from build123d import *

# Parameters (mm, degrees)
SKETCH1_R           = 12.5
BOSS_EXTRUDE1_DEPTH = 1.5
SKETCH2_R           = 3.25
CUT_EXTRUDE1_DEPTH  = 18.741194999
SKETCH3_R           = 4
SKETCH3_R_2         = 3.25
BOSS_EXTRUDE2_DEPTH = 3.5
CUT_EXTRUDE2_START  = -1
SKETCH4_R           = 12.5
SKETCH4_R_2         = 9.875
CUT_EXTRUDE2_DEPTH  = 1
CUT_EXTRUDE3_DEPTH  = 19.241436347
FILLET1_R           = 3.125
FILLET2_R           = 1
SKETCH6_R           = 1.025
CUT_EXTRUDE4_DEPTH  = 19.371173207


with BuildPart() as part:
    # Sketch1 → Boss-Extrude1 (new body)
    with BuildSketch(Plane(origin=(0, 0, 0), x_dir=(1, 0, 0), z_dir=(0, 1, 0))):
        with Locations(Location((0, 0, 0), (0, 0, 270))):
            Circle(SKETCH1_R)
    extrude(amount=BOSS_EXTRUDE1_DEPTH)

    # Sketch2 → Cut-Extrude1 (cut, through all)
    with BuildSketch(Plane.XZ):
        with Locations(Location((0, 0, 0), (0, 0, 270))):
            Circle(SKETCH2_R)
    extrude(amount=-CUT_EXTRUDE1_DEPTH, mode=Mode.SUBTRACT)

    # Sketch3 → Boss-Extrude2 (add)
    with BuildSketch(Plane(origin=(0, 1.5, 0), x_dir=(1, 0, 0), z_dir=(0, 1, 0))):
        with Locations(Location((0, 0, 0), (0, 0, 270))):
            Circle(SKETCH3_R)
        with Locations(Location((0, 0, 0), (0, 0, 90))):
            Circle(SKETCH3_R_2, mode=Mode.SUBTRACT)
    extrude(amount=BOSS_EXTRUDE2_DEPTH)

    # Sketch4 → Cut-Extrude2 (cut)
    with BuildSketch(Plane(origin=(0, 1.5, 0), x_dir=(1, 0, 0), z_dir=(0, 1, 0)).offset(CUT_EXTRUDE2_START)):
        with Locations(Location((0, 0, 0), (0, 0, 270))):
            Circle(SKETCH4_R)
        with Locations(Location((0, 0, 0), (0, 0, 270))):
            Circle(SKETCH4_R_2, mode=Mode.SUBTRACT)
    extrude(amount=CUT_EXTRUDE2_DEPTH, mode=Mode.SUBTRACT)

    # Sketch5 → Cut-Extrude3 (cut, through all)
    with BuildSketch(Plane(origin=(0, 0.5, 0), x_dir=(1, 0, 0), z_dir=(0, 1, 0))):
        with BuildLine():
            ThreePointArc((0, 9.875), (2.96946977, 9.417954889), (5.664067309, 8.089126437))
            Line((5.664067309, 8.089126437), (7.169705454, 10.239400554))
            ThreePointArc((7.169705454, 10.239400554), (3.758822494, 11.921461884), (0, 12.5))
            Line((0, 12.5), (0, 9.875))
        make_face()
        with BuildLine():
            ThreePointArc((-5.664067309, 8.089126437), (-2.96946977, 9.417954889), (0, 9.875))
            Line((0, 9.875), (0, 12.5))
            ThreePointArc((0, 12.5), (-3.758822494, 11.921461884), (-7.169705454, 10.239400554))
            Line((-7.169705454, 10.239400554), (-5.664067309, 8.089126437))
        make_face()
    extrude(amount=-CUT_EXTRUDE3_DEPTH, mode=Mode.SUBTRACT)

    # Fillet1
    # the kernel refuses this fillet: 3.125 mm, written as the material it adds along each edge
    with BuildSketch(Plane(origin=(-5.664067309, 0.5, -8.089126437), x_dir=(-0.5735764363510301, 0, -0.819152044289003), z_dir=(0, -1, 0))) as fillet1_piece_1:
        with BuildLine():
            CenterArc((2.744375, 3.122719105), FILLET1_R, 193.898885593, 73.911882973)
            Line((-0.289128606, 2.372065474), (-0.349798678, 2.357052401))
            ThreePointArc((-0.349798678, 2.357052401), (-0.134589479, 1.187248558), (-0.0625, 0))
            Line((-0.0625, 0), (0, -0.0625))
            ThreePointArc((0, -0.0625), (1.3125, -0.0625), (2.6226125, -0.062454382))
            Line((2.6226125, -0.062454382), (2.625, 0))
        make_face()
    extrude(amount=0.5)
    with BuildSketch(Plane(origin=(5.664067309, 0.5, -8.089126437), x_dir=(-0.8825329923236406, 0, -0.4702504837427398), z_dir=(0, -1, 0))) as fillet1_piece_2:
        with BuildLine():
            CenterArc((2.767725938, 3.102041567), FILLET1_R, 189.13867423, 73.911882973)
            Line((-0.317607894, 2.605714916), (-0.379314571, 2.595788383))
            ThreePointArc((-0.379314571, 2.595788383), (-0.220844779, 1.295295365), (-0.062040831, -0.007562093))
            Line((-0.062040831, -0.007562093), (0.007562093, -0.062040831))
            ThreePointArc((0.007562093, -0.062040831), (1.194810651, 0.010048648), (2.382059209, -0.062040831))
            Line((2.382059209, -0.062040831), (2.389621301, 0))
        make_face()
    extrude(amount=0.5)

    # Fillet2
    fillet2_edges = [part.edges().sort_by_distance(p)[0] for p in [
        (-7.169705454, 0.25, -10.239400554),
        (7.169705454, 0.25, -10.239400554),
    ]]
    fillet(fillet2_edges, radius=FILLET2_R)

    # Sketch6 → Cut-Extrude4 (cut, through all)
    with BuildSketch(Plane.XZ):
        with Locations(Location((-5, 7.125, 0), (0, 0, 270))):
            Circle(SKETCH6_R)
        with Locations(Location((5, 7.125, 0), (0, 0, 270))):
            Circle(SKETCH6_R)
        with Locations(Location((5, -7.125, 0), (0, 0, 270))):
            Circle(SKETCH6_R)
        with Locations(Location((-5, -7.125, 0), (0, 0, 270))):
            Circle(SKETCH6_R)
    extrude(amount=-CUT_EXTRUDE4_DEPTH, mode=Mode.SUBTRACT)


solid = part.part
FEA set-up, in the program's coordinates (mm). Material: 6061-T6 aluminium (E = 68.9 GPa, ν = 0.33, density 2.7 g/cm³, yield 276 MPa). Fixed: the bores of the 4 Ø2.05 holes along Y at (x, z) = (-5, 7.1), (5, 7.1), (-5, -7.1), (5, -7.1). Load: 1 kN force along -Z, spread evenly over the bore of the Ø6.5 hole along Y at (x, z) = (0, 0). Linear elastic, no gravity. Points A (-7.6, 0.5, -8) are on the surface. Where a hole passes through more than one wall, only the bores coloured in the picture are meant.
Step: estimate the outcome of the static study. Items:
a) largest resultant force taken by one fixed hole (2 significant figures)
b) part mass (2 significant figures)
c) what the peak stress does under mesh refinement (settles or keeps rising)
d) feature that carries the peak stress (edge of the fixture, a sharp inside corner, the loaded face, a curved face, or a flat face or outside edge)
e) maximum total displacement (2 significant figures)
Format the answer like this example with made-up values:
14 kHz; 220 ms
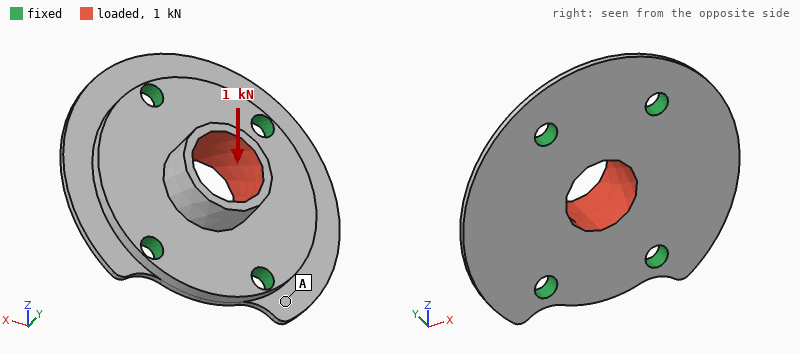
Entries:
270 N; 1.4 g; keeps rising; edge of the fixture; 22 µm
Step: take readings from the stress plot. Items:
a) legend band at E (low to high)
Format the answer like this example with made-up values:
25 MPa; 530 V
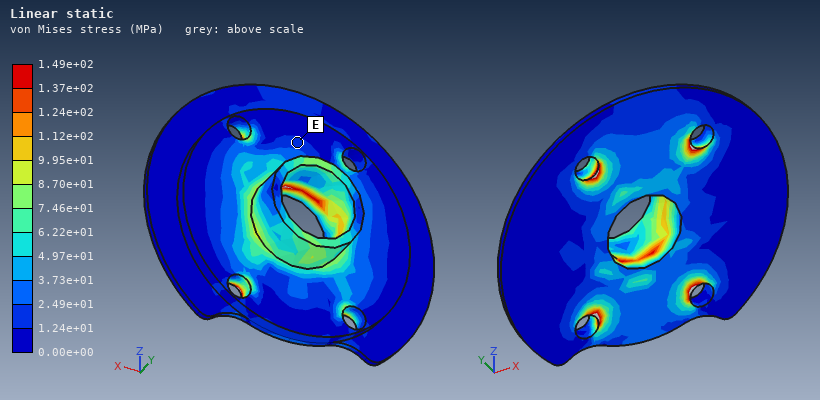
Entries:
1.24e+01 to 2.49e+01 MPa
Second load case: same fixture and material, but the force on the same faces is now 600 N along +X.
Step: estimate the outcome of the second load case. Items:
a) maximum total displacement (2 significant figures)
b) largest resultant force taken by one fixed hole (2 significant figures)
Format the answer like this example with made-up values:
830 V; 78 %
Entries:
17 µm; 170 N
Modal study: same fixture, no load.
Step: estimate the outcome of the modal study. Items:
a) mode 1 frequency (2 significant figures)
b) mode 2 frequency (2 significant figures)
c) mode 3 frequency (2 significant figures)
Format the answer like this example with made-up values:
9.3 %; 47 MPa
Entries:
25 kHz; 25 kHz; 40 kHz
